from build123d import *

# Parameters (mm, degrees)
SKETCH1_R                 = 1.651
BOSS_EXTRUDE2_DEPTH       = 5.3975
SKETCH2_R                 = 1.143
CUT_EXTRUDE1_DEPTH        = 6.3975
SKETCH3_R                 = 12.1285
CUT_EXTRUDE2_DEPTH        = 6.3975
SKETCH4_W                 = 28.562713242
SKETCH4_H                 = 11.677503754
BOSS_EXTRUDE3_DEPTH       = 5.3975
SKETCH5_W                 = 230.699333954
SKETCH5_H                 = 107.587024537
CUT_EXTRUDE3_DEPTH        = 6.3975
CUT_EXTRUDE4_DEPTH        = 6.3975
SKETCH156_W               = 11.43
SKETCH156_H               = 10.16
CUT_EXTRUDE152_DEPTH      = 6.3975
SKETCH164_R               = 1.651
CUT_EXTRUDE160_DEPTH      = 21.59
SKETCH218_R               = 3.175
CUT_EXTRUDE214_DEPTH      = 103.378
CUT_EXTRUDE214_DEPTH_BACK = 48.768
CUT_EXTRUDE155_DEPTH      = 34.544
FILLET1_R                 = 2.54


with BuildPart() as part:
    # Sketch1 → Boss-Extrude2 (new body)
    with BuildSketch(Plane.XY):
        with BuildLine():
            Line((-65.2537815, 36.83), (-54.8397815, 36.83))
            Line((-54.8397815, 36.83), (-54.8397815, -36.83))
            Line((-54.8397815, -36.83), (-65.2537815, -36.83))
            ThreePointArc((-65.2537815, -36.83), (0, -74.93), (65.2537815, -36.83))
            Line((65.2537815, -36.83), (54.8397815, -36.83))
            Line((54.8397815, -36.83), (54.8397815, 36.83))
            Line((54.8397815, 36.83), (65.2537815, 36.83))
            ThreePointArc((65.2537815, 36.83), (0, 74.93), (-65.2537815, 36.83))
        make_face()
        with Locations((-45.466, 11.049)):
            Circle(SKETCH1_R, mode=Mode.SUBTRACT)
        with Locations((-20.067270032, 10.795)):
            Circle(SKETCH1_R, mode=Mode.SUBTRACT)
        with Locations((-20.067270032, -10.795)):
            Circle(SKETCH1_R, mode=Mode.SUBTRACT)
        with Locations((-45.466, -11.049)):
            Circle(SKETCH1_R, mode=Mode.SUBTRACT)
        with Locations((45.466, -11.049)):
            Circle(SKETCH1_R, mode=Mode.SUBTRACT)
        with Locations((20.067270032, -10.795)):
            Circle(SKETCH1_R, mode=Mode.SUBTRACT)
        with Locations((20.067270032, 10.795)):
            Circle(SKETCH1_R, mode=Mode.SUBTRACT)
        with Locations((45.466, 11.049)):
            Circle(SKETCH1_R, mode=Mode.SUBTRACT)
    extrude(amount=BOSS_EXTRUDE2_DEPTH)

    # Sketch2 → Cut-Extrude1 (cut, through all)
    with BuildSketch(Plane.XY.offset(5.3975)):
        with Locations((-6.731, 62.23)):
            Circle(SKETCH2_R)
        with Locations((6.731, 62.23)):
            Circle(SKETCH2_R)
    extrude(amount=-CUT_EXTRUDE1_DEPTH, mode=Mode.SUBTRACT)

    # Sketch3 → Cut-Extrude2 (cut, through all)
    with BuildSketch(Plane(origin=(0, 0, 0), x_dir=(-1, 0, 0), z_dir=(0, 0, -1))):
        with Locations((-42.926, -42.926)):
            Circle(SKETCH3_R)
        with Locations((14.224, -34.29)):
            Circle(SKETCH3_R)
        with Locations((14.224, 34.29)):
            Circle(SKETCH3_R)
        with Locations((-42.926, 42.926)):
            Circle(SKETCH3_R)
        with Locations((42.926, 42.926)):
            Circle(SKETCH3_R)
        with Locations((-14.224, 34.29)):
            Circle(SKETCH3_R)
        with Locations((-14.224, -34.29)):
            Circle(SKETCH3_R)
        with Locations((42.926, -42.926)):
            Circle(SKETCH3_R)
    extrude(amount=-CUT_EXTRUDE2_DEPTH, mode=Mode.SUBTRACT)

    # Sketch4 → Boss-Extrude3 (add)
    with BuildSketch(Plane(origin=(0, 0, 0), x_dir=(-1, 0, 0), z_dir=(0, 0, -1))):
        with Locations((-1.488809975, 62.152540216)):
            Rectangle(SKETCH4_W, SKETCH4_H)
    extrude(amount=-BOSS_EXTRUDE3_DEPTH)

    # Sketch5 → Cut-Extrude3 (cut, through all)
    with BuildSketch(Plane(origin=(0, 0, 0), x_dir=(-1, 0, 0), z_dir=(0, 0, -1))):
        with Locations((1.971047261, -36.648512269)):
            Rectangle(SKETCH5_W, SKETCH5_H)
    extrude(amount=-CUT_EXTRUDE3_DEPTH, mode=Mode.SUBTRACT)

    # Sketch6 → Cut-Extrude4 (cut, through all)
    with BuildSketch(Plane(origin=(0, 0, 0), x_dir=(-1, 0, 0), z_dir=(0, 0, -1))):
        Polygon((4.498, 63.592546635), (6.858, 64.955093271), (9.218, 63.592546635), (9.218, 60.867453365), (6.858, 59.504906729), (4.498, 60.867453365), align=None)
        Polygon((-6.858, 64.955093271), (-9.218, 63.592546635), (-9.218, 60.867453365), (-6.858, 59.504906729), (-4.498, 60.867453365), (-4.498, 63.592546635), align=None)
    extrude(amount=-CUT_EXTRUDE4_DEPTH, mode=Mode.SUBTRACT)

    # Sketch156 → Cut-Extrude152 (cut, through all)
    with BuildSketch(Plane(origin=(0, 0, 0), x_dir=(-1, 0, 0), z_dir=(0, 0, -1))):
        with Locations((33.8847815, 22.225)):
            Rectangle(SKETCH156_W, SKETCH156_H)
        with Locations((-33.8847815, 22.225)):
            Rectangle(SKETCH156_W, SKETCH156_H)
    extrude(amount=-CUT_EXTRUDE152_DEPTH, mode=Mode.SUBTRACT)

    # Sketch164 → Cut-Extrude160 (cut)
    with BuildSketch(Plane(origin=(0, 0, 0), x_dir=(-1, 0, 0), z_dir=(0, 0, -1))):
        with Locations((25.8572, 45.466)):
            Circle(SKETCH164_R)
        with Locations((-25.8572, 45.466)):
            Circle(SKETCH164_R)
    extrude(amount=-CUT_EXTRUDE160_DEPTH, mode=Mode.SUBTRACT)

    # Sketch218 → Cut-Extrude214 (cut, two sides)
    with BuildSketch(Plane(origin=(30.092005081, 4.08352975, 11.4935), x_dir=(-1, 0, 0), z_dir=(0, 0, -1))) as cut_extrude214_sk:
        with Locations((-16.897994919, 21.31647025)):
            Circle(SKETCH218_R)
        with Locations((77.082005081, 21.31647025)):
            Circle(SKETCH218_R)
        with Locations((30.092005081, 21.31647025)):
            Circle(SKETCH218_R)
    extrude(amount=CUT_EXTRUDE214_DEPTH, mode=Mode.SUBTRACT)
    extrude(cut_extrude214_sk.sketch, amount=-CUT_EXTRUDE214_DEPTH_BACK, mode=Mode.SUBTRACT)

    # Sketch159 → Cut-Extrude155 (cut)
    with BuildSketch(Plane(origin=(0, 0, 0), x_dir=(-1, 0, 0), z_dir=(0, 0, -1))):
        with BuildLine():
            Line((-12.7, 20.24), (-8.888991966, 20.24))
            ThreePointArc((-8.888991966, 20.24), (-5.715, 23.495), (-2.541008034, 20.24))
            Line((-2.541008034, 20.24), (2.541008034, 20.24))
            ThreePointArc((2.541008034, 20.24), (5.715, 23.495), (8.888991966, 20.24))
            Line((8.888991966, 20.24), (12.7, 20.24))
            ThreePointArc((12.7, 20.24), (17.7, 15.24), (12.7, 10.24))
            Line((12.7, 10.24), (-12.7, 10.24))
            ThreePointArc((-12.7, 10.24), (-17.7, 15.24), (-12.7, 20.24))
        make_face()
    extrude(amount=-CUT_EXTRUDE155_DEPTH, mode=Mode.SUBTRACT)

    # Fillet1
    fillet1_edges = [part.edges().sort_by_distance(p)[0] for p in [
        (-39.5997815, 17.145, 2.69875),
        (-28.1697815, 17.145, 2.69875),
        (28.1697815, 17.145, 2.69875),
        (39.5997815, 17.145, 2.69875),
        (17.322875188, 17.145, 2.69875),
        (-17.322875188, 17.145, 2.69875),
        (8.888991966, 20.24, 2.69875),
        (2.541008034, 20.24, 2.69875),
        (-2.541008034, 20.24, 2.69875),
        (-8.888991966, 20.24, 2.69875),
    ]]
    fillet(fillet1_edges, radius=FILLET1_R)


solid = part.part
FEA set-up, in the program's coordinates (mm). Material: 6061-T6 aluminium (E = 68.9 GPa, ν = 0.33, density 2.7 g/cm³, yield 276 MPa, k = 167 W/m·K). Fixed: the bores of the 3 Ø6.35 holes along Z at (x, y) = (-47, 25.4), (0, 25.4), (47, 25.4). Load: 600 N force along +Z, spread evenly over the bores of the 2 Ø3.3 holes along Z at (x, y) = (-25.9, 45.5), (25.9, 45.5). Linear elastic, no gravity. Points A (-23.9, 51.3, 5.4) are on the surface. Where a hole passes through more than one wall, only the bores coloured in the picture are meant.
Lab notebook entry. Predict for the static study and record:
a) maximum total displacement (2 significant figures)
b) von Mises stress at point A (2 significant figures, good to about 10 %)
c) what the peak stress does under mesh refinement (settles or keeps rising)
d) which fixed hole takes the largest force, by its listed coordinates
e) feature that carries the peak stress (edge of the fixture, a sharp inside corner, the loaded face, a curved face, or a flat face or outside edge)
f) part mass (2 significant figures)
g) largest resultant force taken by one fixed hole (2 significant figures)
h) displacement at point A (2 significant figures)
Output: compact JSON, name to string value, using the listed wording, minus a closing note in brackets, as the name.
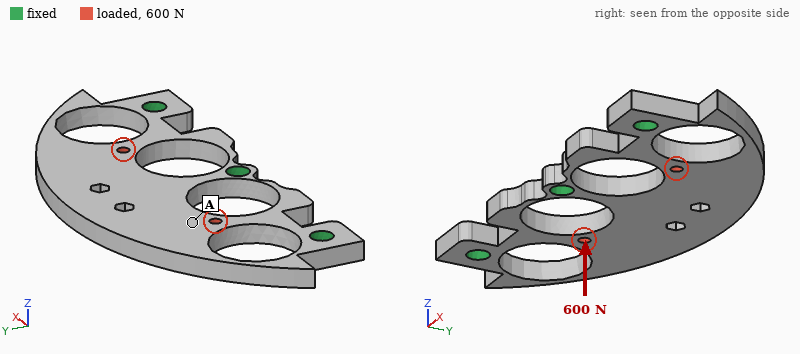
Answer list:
{"maximum total displacement": "0.32 mm", "von Mises stress at point A": "20 MPa", "what the peak stress does under mesh refinement": "keeps rising", "which fixed hole takes the largest force, by its listed coordinates": "(0, 25.4)", "feature that carries the peak stress": "edge of the fixture", "part mass": "48 g", "largest resultant force taken by one fixed hole": "260 N", "displacement at point A": "0.16 mm"}
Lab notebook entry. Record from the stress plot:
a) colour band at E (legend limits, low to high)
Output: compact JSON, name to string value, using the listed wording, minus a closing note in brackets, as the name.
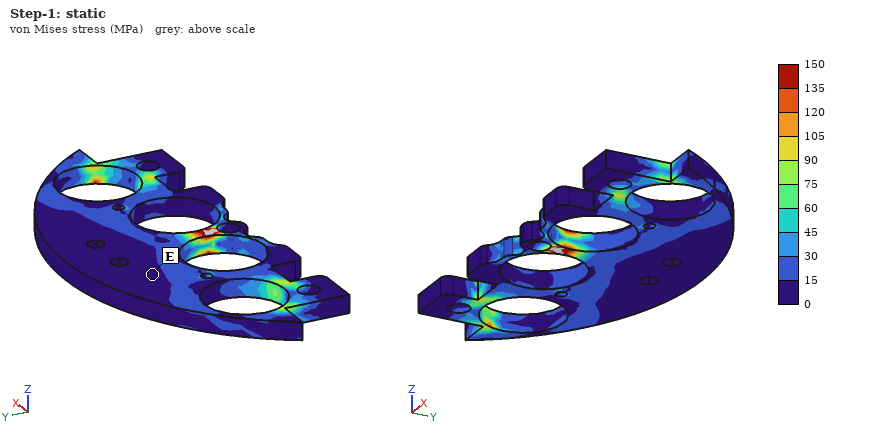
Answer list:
{"colour band at E": "0 to 15 MPa"}
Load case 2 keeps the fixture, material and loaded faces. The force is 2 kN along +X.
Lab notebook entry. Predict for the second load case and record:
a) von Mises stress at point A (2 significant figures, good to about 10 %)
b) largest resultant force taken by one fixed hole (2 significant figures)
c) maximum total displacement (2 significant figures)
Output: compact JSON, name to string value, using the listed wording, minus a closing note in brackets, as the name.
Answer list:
{"von Mises stress at point A": "15 MPa", "largest resultant force taken by one fixed hole": "830 N", "maximum total displacement": "40 µm"}
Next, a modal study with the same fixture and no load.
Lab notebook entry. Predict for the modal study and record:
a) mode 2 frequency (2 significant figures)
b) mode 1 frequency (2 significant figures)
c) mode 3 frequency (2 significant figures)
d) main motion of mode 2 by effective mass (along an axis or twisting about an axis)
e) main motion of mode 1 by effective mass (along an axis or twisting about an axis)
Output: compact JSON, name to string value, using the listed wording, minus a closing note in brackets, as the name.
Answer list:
{"mode 2 frequency": "2700 Hz", "mode 1 frequency": "1000 Hz", "mode 3 frequency": "5400 Hz", "main motion of mode 2 by effective mass": "twisting about Y", "main motion of mode 1 by effective mass": "along Z"}
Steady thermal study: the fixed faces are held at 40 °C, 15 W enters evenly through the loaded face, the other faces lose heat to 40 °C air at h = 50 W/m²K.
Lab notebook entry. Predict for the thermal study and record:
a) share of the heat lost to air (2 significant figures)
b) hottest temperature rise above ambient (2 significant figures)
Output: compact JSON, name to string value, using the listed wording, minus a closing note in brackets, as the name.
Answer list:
{"share of the heat lost to air": "28 %", "hottest temperature rise above ambient": "15 K"}
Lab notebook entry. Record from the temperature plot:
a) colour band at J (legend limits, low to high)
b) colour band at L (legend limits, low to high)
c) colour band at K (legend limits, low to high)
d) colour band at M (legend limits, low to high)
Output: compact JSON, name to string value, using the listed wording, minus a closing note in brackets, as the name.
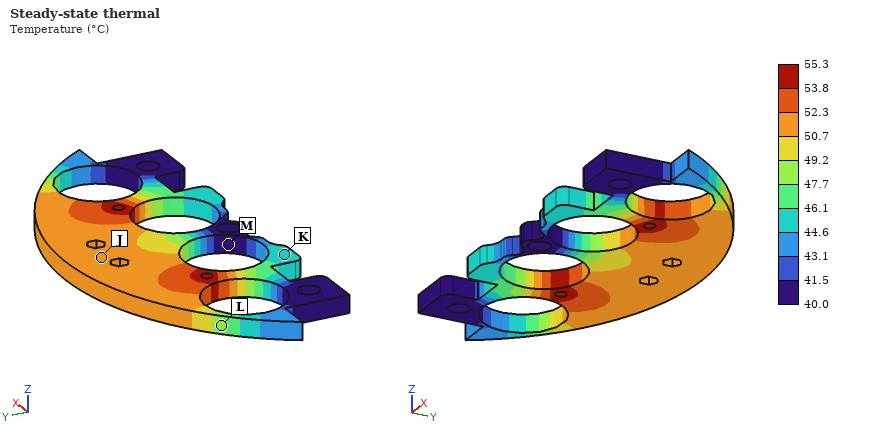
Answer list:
{"colour band at J": "50.7 to 52.3 °C", "colour band at L": "47.7 to 49.2 °C", "colour band at K": "44.6 to 46.1 °C", "colour band at M": "40.0 to 41.5 °C"}
